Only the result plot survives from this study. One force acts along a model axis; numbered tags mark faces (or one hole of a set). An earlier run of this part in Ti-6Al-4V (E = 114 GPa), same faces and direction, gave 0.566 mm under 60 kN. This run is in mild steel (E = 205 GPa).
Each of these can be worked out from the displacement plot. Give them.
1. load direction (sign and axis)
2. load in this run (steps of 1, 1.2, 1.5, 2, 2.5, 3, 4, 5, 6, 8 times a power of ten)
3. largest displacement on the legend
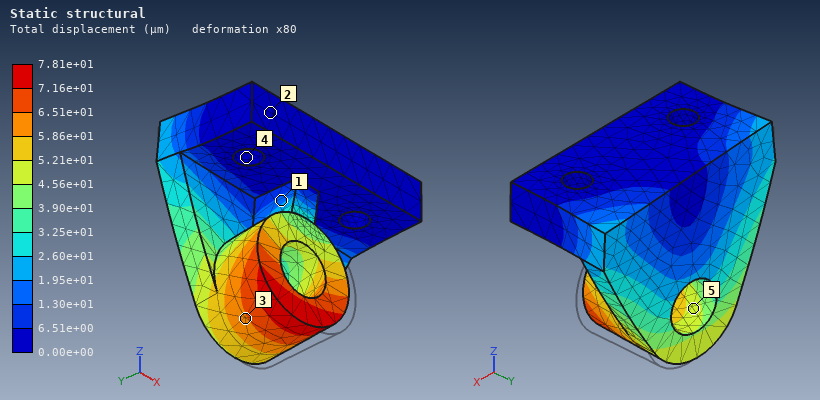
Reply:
-X
15 kN
7.81e+01 µm
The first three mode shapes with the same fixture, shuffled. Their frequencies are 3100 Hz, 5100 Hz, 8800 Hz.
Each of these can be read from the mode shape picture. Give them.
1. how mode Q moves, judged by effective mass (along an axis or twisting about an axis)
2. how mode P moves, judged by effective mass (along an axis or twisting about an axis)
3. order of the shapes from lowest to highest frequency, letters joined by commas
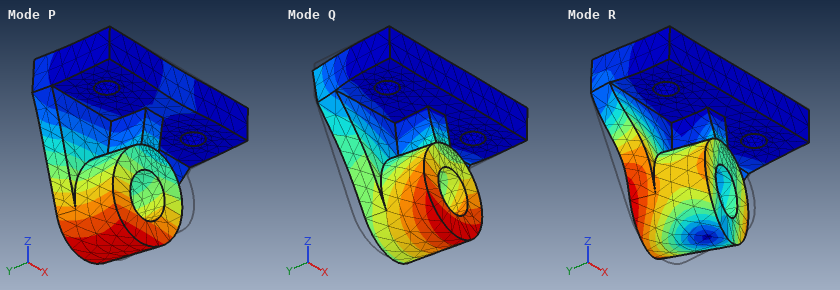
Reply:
along X
along Y
P, Q, R
